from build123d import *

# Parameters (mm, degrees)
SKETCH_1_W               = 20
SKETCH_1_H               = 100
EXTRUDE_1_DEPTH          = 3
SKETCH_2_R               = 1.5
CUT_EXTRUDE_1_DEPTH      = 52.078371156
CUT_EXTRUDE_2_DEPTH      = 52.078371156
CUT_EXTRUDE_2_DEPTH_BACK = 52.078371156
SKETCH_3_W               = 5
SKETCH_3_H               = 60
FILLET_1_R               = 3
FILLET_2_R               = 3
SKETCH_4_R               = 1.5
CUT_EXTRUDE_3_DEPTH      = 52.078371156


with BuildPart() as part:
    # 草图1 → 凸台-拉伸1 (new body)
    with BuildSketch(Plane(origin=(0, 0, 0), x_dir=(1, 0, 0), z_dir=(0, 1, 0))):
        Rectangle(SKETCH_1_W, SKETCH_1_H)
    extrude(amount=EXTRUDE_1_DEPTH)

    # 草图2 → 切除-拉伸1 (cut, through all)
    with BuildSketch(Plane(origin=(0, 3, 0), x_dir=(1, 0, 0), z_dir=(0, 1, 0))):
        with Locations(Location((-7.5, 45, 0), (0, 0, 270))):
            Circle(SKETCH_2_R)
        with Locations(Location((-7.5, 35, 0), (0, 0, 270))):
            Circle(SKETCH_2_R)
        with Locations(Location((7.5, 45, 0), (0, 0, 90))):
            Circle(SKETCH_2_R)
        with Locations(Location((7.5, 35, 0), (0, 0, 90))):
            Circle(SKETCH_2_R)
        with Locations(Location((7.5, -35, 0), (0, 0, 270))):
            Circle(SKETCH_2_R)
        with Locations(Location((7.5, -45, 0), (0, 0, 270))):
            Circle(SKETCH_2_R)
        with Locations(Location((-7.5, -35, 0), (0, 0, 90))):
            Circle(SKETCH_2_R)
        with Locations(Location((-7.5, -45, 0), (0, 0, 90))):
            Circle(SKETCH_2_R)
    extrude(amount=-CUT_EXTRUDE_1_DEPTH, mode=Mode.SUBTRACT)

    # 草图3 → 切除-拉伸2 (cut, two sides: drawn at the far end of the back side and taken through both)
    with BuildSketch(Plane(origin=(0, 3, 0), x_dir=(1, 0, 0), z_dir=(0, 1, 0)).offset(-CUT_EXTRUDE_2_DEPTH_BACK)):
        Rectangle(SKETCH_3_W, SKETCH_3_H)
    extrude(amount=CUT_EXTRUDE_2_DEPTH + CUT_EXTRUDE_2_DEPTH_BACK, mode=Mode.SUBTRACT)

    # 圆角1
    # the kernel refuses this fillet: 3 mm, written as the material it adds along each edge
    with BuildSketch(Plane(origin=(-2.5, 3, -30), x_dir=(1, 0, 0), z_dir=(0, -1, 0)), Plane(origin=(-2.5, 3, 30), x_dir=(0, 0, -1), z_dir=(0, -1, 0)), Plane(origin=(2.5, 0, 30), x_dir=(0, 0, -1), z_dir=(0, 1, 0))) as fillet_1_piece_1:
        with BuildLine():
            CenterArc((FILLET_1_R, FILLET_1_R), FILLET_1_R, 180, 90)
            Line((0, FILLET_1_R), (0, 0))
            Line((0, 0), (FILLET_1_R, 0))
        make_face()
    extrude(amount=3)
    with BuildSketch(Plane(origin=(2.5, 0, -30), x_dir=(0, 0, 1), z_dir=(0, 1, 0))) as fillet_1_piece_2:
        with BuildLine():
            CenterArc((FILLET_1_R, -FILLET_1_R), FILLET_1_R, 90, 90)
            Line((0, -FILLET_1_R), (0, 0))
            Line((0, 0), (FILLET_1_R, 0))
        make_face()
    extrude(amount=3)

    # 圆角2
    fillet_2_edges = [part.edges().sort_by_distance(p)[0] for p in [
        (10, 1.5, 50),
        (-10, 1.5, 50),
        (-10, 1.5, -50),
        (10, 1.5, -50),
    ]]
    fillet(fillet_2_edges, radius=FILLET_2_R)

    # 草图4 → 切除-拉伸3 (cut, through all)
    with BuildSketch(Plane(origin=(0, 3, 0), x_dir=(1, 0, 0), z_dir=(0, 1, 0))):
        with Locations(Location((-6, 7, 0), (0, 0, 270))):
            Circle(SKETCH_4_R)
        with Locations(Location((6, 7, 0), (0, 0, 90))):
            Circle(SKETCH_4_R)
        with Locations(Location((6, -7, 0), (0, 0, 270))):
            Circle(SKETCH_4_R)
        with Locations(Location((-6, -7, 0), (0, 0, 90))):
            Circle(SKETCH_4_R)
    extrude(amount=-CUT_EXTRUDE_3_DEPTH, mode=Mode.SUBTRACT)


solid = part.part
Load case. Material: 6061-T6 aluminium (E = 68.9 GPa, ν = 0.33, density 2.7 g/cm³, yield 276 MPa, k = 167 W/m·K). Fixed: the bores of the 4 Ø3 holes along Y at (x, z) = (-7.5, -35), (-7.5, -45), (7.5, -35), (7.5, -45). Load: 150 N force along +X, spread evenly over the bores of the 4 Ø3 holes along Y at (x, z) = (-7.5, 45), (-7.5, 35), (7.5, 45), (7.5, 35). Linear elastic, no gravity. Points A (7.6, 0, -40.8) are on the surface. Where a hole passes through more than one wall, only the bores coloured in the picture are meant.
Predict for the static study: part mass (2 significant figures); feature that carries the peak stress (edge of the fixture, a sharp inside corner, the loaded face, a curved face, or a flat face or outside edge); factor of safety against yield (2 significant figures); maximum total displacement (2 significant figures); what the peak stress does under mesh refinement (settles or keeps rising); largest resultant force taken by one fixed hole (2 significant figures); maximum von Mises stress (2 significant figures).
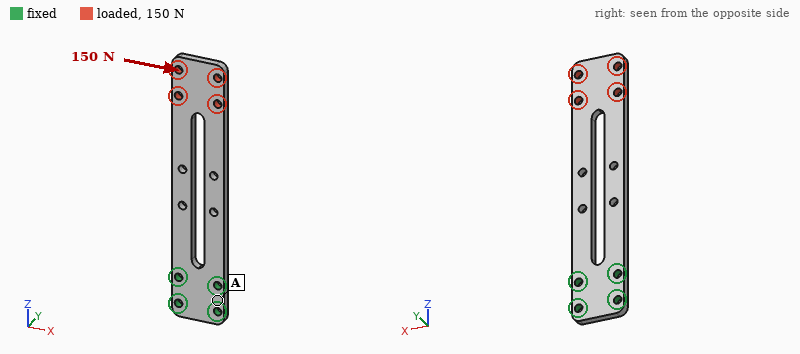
13 g
a curved face
2.4
0.40 mm
settles
690 N
110 MPa
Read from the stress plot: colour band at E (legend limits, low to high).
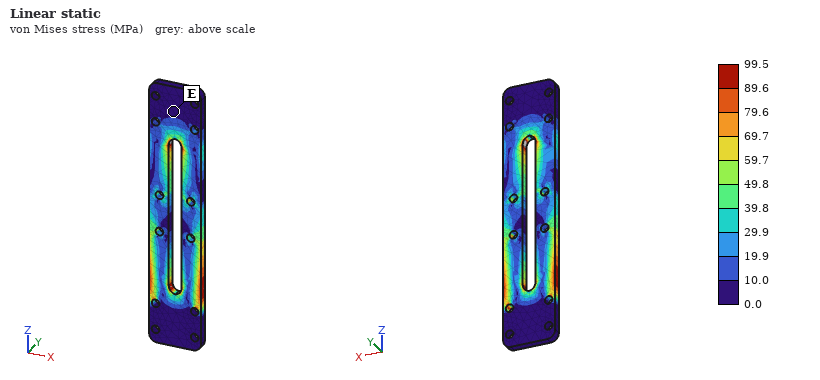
0.0 to 10.0 MPa
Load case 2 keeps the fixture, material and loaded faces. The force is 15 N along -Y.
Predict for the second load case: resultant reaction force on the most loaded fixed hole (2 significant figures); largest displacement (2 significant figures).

20 N
1.1 mm
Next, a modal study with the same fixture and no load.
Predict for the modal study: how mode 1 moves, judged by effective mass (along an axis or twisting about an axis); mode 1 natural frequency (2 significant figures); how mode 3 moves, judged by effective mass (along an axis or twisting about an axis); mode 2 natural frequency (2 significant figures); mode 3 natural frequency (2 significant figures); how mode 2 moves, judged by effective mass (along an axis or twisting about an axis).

along Y
320 Hz
along Y
1400 Hz
2100 Hz
along X
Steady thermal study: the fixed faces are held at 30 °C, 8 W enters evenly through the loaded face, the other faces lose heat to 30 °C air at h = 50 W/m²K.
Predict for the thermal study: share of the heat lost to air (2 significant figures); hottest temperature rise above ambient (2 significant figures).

56 %
47 K
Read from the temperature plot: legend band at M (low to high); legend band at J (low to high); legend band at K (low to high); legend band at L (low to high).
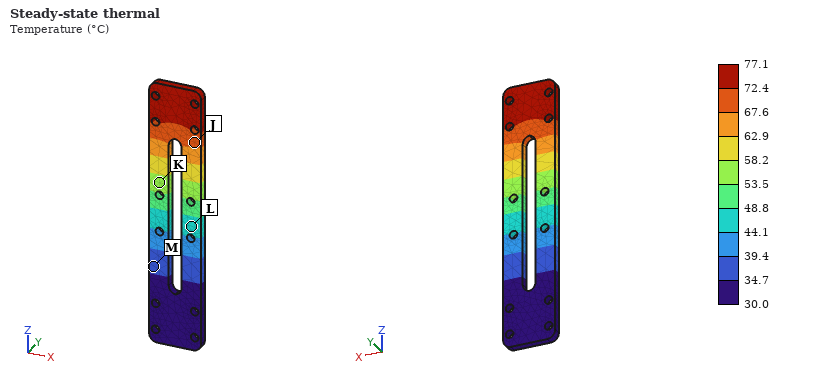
34.7 to 39.4 °C
67.6 to 72.4 °C
53.5 to 58.2 °C
44.1 to 48.8 °C
